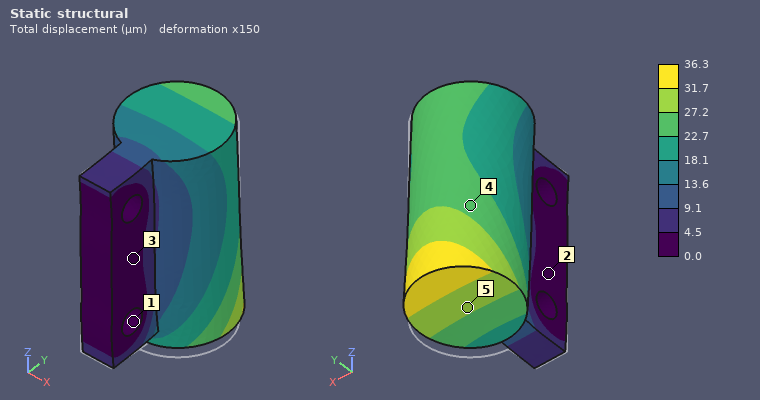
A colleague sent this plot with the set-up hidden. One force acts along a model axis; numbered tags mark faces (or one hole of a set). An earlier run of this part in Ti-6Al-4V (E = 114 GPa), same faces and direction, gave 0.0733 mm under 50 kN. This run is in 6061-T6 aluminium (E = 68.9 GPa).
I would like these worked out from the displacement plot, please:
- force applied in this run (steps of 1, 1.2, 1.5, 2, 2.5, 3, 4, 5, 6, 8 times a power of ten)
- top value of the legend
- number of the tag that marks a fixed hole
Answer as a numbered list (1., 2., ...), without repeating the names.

1. 15 kN
2. 36.3 µm
3. 1
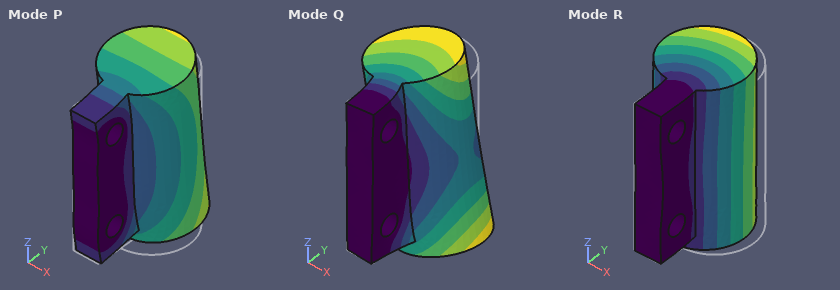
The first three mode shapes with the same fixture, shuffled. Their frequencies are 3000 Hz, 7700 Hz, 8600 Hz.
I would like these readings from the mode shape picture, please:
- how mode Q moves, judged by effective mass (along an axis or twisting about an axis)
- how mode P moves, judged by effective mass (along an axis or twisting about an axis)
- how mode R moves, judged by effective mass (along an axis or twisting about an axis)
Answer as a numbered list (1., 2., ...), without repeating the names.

1. twisting about Y
2. along Z
3. along X
